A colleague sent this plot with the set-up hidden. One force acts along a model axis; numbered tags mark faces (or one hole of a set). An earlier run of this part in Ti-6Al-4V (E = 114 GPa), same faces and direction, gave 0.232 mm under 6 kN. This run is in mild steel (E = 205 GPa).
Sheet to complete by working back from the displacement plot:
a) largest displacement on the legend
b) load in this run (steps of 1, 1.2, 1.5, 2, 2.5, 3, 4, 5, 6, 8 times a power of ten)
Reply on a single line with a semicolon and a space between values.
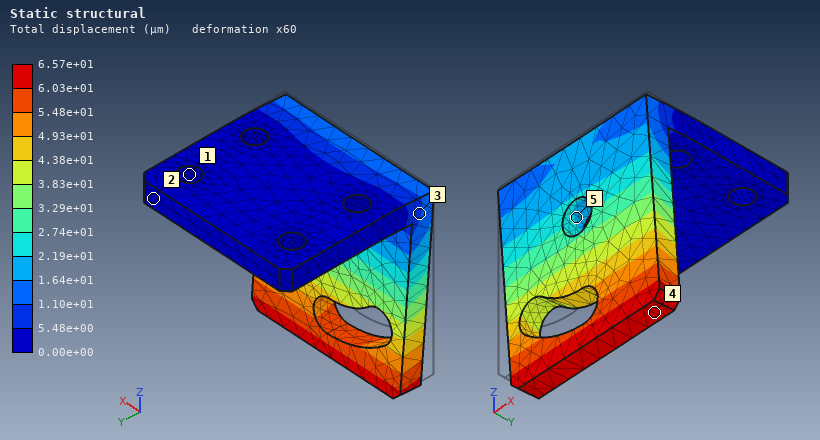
6.57e+01 µm; 3 kN
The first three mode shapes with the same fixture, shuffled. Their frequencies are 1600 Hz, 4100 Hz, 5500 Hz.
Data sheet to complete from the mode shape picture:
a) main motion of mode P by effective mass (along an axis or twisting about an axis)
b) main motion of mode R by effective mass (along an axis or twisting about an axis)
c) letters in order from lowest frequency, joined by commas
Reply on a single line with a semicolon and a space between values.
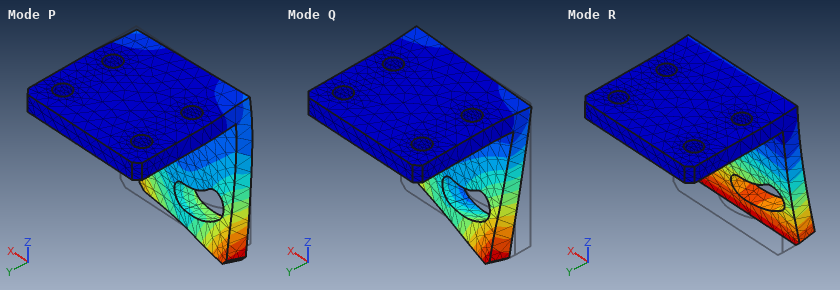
along X; along Y; R, Q, P
